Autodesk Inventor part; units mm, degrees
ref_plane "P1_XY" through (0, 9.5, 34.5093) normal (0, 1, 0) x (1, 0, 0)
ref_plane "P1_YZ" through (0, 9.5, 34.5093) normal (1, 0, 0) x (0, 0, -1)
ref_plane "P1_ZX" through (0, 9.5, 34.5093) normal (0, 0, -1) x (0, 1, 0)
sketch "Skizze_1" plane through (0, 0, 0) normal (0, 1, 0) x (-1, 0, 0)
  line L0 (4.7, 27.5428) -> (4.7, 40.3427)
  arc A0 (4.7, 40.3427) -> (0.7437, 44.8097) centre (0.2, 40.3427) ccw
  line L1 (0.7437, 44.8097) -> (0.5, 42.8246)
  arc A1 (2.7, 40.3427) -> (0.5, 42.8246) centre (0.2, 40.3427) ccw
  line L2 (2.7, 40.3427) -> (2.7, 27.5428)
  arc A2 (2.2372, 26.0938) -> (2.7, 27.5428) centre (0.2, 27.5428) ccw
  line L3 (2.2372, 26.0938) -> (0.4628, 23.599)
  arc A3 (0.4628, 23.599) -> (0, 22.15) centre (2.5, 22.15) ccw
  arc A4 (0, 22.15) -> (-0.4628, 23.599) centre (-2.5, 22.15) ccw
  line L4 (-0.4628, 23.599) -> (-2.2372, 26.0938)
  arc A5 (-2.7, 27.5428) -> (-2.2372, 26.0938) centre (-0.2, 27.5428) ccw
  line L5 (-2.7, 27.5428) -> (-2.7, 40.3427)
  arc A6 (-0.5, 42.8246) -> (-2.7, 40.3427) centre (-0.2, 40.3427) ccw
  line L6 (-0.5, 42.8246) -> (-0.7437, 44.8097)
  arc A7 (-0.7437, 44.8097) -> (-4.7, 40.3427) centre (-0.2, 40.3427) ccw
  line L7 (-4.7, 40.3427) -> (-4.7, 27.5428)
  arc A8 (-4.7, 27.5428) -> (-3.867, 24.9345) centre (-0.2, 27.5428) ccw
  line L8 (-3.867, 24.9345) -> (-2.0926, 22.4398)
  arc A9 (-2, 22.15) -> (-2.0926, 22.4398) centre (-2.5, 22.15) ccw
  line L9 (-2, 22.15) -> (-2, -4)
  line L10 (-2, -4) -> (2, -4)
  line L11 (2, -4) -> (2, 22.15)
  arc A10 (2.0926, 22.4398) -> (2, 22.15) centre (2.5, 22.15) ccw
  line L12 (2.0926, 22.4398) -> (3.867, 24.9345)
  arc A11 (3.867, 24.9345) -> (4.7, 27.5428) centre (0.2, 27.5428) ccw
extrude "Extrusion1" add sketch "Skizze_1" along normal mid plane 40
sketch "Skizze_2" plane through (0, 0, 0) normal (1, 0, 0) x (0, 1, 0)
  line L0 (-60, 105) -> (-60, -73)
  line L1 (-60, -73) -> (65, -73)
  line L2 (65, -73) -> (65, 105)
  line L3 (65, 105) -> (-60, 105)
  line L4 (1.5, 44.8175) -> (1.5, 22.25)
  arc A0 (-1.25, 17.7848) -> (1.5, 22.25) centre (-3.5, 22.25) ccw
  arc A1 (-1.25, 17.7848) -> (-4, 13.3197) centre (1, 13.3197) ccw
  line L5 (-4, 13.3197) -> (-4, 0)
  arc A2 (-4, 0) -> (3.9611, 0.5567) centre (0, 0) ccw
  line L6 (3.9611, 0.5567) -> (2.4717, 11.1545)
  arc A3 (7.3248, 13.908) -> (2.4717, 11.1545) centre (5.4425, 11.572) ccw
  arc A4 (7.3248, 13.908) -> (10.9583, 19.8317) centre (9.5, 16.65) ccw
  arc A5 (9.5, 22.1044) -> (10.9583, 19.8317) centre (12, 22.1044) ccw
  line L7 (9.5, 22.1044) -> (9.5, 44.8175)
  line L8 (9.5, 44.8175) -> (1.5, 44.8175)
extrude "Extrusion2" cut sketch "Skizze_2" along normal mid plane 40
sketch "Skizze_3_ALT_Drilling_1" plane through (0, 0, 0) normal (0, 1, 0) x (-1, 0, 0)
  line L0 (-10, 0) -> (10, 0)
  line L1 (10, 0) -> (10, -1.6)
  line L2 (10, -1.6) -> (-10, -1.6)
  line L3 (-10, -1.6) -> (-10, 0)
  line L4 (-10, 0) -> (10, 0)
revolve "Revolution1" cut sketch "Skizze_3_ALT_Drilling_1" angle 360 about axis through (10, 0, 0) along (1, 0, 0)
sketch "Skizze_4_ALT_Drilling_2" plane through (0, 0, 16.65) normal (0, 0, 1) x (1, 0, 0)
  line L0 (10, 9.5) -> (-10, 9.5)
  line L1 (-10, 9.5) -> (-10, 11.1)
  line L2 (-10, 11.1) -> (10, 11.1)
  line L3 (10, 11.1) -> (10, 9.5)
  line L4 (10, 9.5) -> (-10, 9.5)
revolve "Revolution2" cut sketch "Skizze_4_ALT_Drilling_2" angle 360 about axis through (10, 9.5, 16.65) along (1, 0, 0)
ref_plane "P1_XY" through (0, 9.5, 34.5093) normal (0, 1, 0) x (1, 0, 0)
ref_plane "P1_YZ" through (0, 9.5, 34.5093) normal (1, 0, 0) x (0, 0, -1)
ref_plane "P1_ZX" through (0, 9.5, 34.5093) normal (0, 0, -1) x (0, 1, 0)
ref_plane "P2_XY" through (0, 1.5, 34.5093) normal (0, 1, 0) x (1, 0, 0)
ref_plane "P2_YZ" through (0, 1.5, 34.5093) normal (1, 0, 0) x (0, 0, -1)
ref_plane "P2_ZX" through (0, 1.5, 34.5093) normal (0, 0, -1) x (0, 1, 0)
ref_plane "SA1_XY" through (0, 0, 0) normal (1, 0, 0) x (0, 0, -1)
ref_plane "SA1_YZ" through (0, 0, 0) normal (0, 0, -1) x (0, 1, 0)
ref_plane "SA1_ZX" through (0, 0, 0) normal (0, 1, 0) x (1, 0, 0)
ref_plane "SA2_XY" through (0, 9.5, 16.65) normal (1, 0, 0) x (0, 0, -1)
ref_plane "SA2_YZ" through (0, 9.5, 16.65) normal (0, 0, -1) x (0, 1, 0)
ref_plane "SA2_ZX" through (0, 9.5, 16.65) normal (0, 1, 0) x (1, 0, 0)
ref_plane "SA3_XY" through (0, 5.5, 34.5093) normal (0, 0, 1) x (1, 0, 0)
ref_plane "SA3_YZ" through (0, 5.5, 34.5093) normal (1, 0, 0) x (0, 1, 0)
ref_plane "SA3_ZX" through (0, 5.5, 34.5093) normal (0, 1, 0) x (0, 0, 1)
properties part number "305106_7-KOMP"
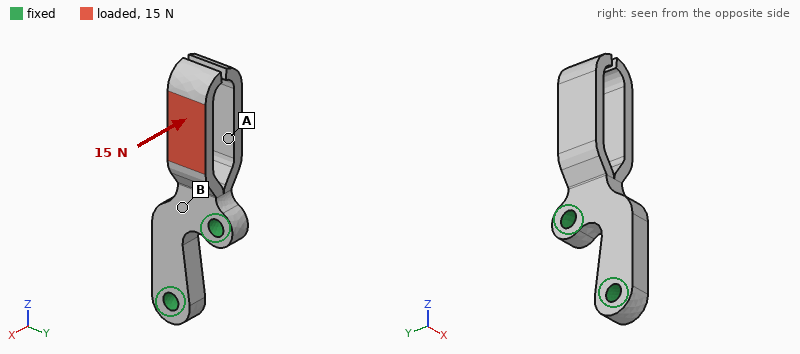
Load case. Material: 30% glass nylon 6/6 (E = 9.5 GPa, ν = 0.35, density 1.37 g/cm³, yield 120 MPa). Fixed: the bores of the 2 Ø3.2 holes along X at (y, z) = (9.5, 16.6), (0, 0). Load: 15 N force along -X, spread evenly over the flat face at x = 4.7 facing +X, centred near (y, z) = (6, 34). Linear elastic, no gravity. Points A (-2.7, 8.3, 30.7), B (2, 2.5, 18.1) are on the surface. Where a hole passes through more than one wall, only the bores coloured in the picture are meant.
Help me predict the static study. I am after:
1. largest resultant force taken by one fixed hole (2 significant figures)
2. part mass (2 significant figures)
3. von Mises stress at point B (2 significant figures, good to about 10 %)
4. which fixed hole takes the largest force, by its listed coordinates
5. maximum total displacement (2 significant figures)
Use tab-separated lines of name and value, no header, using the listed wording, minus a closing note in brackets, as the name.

largest resultant force taken by one fixed hole	19 N
part mass	2.2 g
von Mises stress at point B	5.1 MPa
which fixed hole takes the largest force, by its listed coordinates	(9.5, 16.6)
maximum total displacement	0.57 mm
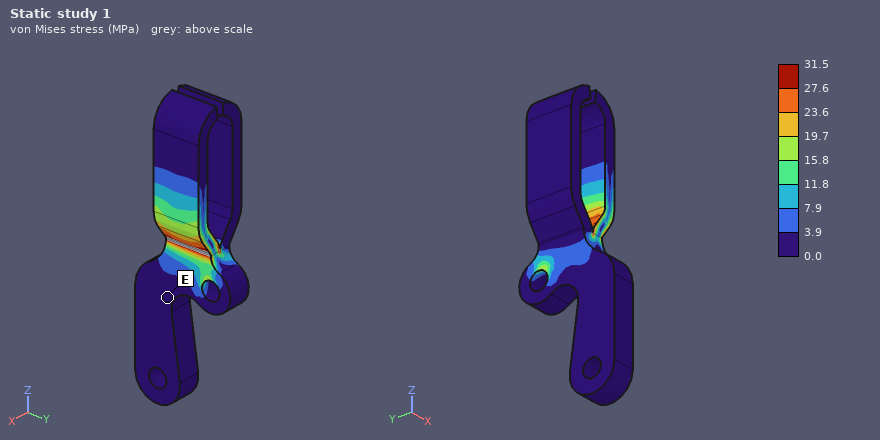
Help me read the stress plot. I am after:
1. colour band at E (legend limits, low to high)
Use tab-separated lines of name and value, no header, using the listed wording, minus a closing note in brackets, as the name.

colour band at E	0.0 to 3.9 MPa
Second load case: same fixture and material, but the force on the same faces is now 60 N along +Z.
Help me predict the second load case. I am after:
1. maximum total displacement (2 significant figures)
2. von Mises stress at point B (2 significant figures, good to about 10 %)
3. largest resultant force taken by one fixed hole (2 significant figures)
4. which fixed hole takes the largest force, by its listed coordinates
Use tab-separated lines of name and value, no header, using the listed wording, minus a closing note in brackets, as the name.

maximum total displacement	0.58 mm
von Mises stress at point B	7.7 MPa
largest resultant force taken by one fixed hole	41 N
which fixed hole takes the largest force, by its listed coordinates	(9.5, 16.6)
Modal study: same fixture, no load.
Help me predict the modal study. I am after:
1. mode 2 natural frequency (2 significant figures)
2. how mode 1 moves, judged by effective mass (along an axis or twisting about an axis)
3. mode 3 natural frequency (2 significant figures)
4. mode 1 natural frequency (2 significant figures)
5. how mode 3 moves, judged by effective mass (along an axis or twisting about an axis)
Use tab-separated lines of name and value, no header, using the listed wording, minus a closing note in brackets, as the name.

mode 2 natural frequency	1400 Hz
how mode 1 moves, judged by effective mass	along X
mode 3 natural frequency	3400 Hz
mode 1 natural frequency	1300 Hz
how mode 3 moves, judged by effective mass	along Y
